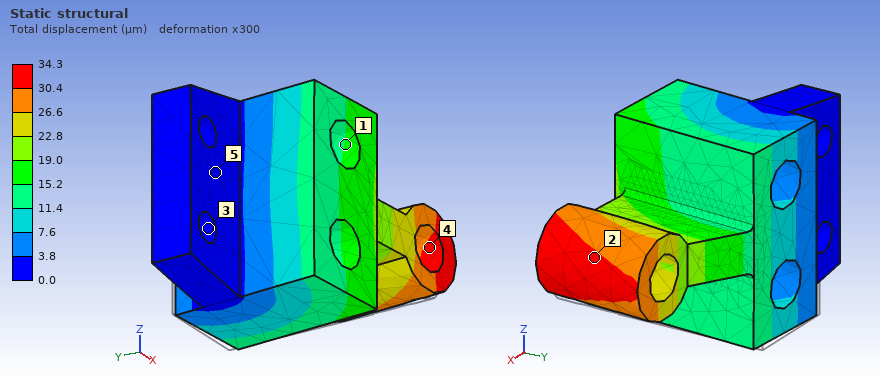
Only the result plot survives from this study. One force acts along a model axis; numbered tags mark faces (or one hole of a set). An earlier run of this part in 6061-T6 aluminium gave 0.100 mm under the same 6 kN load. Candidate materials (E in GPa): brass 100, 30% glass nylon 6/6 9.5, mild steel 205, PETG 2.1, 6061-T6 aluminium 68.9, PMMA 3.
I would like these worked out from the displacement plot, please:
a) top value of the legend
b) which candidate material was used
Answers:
34.3 µm
mild steel
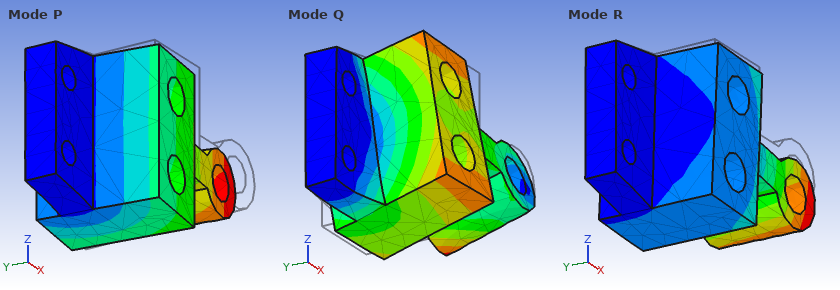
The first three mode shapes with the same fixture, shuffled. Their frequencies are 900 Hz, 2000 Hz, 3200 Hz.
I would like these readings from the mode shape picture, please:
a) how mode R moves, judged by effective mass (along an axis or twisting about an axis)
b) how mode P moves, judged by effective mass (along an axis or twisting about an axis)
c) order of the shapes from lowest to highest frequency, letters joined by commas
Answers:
along Z
along Y
P, R, Q
